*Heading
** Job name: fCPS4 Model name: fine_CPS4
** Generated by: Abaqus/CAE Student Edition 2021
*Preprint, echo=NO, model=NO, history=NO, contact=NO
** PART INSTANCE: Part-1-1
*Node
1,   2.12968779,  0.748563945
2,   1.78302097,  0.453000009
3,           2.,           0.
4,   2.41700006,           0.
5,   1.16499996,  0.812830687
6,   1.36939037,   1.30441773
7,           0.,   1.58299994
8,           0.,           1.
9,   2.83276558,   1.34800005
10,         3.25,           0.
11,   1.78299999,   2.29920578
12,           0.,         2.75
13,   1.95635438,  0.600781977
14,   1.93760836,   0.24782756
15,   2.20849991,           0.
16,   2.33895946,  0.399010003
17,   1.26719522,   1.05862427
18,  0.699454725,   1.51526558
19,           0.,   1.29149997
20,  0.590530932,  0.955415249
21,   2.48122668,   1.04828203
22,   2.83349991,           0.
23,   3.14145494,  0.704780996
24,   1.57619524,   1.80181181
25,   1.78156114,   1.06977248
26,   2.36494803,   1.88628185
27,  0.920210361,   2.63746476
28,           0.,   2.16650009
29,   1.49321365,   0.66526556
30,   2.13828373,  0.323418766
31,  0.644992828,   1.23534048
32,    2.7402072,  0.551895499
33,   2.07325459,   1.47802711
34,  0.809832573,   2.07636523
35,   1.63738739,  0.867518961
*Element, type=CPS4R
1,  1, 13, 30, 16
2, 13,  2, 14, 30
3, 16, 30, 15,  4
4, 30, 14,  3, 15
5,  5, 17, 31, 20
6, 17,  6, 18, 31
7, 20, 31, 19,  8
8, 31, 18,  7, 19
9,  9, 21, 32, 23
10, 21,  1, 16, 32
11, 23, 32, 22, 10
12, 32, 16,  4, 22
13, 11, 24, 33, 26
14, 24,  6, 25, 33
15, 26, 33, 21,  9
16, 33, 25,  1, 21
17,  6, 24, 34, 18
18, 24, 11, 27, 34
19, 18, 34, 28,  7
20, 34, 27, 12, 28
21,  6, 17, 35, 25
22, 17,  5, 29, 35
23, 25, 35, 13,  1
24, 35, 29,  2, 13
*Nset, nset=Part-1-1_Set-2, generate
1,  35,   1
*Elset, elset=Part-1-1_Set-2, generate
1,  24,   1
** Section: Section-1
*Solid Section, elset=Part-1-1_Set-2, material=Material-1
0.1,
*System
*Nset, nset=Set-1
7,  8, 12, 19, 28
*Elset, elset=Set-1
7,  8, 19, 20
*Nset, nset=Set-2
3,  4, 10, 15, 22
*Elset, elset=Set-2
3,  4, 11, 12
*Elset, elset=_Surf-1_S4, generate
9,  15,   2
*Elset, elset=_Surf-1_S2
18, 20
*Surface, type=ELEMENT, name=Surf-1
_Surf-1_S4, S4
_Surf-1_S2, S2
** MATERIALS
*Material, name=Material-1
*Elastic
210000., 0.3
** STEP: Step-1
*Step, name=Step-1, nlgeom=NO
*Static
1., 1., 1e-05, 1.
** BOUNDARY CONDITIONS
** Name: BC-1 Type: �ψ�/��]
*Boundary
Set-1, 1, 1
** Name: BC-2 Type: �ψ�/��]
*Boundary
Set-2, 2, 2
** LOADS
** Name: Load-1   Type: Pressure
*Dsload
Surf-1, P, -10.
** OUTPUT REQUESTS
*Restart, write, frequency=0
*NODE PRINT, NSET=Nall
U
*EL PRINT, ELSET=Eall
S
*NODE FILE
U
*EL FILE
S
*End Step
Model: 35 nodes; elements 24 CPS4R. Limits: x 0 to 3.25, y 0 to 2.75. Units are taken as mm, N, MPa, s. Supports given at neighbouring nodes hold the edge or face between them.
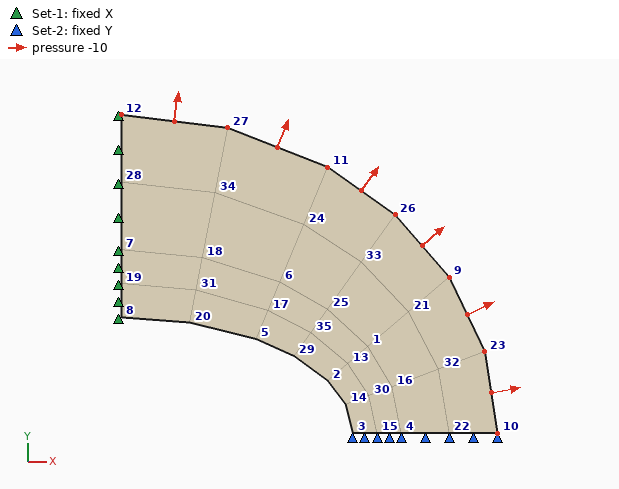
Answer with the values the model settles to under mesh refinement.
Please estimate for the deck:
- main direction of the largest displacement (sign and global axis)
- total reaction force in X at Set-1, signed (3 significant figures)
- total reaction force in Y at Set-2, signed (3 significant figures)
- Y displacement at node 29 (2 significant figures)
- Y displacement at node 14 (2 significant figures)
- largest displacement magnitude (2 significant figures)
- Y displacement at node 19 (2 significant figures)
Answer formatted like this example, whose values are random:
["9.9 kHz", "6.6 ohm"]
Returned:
["+Y", "-2.75 N", "-3.25 N", "3.2e-04 mm", "1.1e-04 mm", "5.5e-04 mm", "5.5e-04 mm"]
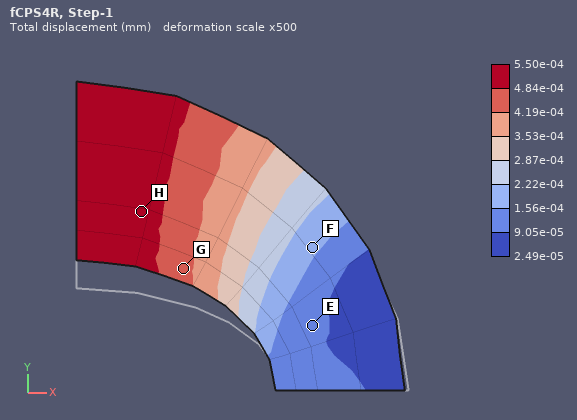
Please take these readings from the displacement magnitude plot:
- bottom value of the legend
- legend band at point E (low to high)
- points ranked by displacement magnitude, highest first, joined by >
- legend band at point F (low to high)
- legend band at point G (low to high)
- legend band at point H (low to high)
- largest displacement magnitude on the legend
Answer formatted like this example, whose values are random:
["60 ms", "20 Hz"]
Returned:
["2.49e-05 mm", "9.05e-05 to 1.56e-04 mm", "H > G > F > E", "1.56e-04 to 2.22e-04 mm", "4.19e-04 to 4.84e-04 mm", "4.84e-04 to 5.50e-04 mm", "5.50e-04 mm"]
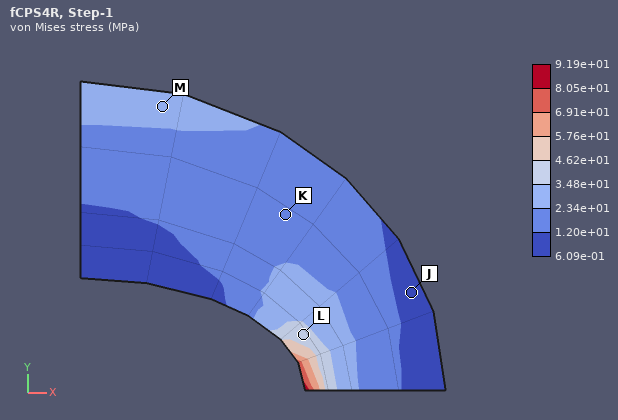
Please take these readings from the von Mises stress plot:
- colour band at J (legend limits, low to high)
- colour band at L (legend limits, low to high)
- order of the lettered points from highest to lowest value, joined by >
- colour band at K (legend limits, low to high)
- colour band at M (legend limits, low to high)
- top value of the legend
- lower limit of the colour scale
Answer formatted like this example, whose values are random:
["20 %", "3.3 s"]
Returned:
["6.09e-01 to 1.20e+01 MPa", "3.48e+01 to 4.62e+01 MPa", "L > M > K > J", "1.20e+01 to 2.34e+01 MPa", "2.34e+01 to 3.48e+01 MPa", "9.19e+01 MPa", "6.09e-01 MPa"]
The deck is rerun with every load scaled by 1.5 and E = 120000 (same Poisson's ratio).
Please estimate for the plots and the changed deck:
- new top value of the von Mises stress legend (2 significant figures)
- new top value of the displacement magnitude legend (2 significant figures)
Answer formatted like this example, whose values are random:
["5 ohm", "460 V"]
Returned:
["140 MPa", "0.0014 mm"]
